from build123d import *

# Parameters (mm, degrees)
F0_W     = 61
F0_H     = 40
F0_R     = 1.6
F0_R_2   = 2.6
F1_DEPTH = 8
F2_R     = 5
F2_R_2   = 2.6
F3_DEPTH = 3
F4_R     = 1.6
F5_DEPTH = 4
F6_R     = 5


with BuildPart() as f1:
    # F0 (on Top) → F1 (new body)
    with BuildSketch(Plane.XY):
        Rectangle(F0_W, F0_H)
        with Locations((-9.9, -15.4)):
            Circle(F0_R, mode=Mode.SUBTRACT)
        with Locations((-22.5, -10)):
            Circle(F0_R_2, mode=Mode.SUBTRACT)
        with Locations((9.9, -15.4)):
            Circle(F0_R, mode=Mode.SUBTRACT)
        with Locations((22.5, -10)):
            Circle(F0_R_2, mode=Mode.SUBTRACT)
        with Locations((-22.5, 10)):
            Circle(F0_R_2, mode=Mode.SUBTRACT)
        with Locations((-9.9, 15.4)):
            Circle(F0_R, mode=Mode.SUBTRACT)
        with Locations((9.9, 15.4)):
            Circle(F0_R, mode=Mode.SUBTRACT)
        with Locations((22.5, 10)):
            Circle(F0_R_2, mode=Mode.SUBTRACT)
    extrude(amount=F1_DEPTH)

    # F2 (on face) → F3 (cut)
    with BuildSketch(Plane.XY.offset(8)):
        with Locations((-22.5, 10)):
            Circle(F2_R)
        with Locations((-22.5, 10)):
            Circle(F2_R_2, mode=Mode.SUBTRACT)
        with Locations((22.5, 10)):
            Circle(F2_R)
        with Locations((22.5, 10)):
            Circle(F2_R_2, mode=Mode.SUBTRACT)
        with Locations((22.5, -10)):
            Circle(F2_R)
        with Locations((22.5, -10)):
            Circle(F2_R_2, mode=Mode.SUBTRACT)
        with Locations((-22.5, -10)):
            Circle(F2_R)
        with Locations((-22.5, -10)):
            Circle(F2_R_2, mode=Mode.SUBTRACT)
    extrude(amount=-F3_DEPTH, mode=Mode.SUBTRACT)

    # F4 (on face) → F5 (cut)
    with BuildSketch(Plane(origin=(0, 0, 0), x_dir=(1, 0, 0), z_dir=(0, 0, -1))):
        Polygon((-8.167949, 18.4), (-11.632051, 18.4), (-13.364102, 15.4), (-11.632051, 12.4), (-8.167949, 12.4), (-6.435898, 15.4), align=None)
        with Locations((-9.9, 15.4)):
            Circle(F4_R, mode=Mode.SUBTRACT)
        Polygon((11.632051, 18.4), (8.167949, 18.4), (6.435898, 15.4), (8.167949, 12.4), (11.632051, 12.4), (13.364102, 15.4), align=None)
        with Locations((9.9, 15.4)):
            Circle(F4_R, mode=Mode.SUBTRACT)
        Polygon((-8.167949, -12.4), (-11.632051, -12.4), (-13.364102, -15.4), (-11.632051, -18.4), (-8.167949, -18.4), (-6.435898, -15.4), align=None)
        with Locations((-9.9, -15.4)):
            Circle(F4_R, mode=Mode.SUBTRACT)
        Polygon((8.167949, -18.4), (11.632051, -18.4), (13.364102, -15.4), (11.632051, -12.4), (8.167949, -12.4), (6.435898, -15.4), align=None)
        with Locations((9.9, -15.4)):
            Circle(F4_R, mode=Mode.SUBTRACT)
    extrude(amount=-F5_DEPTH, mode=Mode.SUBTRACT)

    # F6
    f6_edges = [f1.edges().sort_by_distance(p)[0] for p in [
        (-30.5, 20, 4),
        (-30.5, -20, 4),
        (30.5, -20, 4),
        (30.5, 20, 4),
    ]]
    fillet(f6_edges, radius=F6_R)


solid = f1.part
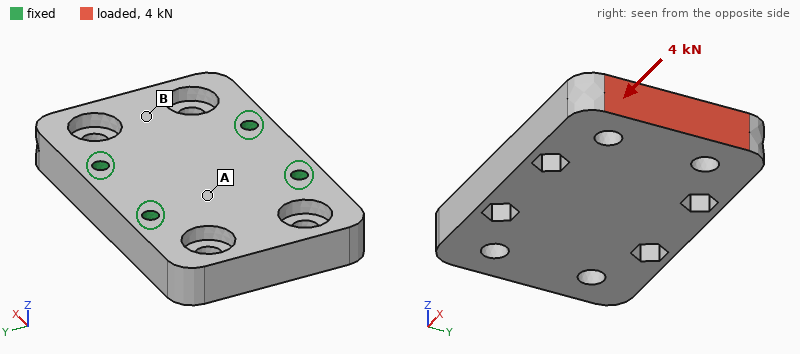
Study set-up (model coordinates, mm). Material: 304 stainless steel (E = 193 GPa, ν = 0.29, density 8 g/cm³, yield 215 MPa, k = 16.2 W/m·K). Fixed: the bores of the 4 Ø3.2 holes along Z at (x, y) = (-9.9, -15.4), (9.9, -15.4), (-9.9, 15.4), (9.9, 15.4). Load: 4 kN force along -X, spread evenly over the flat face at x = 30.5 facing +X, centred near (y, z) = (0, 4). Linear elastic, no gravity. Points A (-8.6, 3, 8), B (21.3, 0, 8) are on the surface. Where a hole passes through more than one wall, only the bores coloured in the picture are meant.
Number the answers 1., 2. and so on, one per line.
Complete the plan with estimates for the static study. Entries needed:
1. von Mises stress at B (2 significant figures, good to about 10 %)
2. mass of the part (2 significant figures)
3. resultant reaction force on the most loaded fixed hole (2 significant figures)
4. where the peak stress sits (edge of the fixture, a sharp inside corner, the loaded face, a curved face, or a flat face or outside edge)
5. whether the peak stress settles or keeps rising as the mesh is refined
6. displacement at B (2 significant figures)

1. 21 MPa
2. 140 g
3. 1.3 kN
4. edge of the fixture
5. keeps rising
6. 2.5 µm
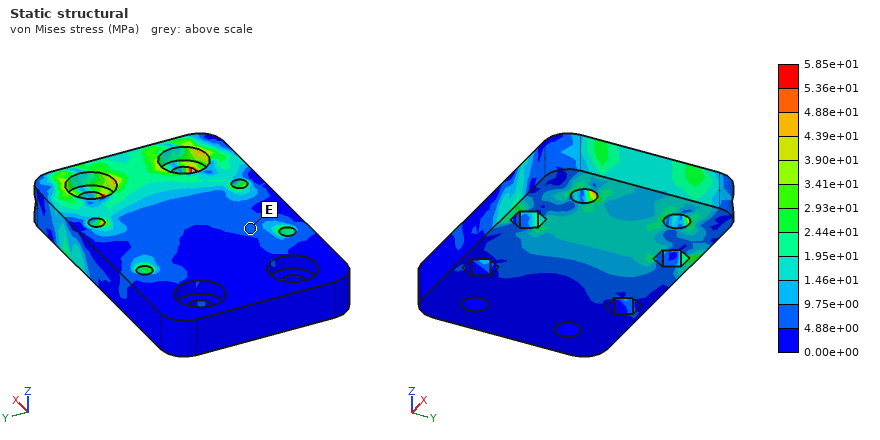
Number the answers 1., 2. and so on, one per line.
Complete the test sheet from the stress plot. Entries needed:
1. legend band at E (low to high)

1. 4.88e+00 to 9.75e+00 MPa
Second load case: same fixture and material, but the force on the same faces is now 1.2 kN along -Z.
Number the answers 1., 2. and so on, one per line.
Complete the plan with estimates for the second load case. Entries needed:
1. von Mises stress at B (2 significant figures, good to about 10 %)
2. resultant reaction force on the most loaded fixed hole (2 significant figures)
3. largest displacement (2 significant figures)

1. 40 MPa
2. 1.3 kN
3. 29 µm
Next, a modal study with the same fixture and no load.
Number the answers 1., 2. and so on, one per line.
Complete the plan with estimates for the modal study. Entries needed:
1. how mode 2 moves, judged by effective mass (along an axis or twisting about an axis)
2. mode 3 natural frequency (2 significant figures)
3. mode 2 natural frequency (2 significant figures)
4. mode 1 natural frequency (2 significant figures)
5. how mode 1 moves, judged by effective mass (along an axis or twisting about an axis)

1. along Z
2. 16 kHz
3. 9500 Hz
4. 8900 Hz
5. twisting about Y
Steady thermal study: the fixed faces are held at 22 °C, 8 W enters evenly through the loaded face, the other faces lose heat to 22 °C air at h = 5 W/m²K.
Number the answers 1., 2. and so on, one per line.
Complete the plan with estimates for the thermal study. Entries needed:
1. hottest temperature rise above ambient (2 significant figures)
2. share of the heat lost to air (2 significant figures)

1. 53 K
2. 5.0 %
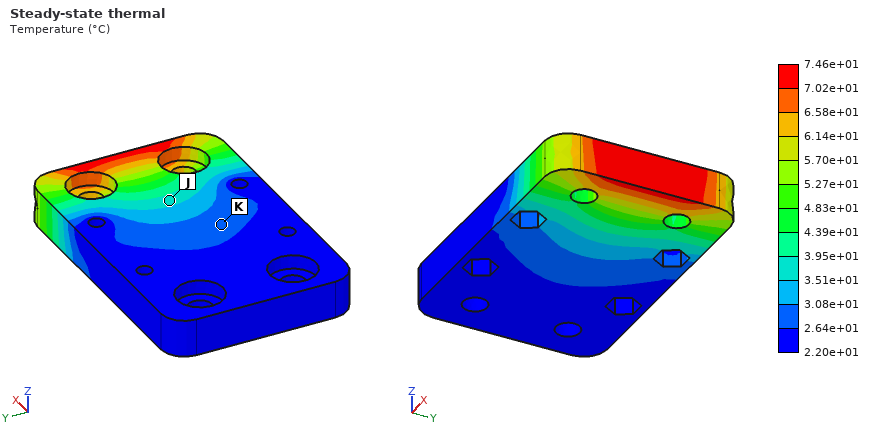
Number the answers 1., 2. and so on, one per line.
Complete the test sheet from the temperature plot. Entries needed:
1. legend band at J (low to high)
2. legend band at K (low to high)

1. 3.51e+01 to 3.95e+01 °C
2. 2.64e+01 to 3.08e+01 °C
